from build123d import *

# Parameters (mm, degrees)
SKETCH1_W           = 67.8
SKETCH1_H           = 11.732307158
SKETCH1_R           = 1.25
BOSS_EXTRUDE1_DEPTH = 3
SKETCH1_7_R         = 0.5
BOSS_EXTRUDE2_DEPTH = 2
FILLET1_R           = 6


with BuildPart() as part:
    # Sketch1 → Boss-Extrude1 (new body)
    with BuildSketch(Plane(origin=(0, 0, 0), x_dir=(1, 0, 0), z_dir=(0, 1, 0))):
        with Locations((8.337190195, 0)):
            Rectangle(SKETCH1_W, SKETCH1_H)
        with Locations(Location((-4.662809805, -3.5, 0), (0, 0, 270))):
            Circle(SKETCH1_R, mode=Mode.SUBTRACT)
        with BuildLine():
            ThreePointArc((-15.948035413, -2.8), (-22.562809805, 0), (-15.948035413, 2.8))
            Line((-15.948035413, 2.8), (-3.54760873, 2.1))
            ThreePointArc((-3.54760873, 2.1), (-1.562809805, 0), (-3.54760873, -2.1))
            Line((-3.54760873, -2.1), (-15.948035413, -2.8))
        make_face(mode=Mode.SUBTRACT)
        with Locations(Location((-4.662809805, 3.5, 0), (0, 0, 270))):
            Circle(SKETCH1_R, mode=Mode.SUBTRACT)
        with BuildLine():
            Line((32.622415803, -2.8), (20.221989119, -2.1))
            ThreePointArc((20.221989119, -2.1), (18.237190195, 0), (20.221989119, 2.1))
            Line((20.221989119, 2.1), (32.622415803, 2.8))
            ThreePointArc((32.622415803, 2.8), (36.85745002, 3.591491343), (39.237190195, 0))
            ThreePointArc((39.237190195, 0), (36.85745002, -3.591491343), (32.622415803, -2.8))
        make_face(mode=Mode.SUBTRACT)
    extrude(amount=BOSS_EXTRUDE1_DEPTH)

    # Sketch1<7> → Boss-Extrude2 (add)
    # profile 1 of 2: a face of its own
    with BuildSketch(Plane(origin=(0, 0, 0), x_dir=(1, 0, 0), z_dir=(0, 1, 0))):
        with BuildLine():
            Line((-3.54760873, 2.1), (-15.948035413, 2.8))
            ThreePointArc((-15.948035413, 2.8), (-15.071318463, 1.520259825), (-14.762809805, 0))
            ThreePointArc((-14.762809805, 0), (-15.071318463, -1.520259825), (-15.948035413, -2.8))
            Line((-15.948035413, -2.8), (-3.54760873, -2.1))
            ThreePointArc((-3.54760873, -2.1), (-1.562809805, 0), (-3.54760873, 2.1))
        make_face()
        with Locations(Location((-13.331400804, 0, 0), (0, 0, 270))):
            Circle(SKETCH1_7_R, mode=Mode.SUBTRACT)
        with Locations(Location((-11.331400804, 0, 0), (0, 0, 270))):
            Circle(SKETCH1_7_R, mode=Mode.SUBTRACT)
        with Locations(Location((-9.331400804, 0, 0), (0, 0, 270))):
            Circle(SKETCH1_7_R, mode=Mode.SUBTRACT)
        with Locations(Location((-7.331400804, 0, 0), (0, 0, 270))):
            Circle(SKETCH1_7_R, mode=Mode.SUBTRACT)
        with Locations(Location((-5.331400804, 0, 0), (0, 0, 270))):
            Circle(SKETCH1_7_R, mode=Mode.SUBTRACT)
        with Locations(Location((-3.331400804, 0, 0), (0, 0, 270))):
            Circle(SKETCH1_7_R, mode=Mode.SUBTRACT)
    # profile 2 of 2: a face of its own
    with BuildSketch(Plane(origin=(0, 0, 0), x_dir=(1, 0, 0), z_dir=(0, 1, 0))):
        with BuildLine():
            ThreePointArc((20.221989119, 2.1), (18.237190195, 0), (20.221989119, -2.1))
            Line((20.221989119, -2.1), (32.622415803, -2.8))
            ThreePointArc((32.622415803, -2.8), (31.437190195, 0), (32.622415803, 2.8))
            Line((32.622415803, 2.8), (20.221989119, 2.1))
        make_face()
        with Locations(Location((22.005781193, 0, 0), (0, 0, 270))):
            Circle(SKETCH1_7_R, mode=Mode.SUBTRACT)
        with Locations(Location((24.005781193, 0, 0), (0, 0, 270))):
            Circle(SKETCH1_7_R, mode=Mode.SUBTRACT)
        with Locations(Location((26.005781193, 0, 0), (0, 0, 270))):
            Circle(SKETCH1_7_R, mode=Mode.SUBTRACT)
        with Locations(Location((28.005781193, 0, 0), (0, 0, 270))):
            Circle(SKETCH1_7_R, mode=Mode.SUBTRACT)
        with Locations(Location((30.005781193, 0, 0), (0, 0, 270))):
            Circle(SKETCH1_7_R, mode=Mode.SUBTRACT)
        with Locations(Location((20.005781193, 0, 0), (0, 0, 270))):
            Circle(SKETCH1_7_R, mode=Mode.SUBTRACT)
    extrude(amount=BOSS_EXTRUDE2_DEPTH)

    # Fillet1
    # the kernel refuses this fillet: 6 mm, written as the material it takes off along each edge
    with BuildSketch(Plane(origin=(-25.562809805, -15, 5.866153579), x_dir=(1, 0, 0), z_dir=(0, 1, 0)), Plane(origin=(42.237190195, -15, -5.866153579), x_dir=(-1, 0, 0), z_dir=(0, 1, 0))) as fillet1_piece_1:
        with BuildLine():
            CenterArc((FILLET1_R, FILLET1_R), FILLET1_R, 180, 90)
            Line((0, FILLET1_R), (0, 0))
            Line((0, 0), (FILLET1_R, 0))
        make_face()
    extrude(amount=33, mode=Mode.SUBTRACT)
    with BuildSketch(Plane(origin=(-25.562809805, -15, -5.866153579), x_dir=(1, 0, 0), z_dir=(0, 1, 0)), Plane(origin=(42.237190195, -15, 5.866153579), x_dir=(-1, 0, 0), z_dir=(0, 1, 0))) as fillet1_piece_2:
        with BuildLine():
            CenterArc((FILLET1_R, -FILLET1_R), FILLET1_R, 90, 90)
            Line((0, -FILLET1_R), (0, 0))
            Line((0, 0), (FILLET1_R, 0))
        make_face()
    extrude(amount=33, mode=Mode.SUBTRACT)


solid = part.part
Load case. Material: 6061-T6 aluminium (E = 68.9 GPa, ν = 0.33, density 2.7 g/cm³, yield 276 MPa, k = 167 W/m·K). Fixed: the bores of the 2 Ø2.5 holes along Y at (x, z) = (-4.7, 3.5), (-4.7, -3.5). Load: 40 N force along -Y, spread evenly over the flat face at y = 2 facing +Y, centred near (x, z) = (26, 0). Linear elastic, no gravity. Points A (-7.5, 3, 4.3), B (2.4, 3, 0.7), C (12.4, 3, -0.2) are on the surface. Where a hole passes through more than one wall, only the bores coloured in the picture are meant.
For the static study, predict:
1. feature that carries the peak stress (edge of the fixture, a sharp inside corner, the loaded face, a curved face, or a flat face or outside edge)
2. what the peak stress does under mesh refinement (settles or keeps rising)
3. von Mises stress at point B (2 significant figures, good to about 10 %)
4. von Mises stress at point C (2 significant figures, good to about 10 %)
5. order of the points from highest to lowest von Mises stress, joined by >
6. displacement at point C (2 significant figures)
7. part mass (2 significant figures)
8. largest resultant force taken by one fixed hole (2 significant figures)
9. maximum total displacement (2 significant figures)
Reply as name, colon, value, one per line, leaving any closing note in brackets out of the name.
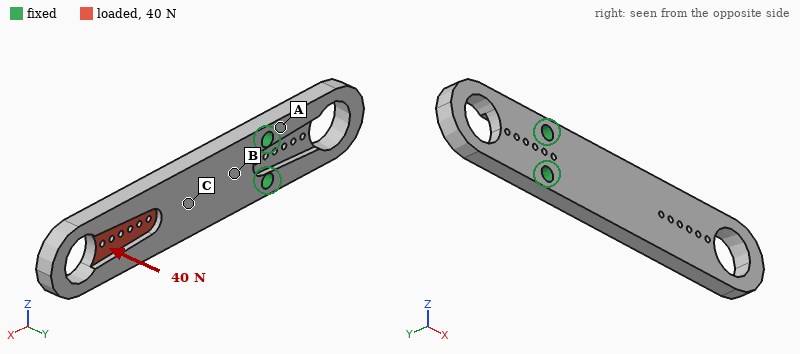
feature that carries the peak stress: edge of the fixture
what the peak stress does under mesh refinement: keeps rising
von Mises stress at point B: 48 MPa
von Mises stress at point C: 30 MPa
order of the points from highest to lowest von Mises stress, joined by >: B > C > A
displacement at point C: 0.078 mm
part mass: 5.0 g
largest resultant force taken by one fixed hole: 20 N
maximum total displacement: 0.37 mm
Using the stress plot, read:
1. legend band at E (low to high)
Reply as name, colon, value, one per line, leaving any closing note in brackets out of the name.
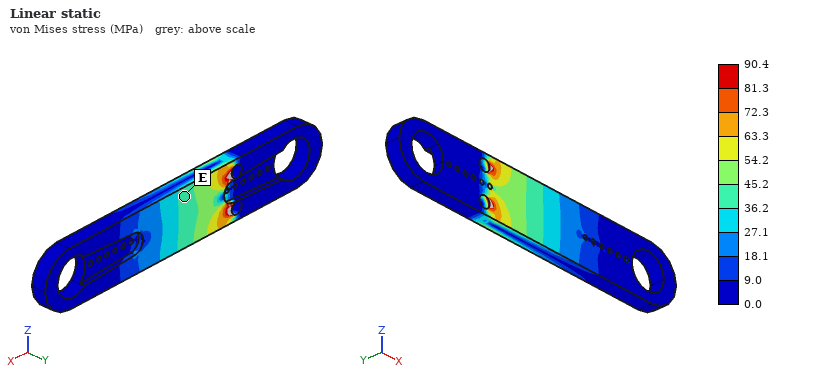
legend band at E: 36.2 to 45.2 MPa
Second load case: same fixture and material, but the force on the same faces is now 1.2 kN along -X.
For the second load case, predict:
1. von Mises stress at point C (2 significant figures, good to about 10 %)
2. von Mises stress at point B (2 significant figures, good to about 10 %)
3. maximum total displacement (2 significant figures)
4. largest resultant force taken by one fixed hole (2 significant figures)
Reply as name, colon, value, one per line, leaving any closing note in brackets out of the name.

von Mises stress at point C: 66 MPa
von Mises stress at point B: 63 MPa
maximum total displacement: 0.36 mm
largest resultant force taken by one fixed hole: 610 N
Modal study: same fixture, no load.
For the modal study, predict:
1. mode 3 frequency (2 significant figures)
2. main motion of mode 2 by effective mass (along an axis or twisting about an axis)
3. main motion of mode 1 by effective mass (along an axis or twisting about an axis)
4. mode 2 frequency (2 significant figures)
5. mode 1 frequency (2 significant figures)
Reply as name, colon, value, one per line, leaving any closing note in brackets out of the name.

mode 3 frequency: 6800 Hz
main motion of mode 2 by effective mass: along Z
main motion of mode 1 by effective mass: along Y
mode 2 frequency: 5200 Hz
mode 1 frequency: 1400 Hz
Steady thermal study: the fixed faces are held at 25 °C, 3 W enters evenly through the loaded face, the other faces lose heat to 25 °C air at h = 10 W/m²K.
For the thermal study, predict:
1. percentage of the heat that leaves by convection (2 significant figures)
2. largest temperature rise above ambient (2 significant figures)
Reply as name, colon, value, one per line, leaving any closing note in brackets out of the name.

percentage of the heat that leaves by convection: 4.4 %
largest temperature rise above ambient: 16 K
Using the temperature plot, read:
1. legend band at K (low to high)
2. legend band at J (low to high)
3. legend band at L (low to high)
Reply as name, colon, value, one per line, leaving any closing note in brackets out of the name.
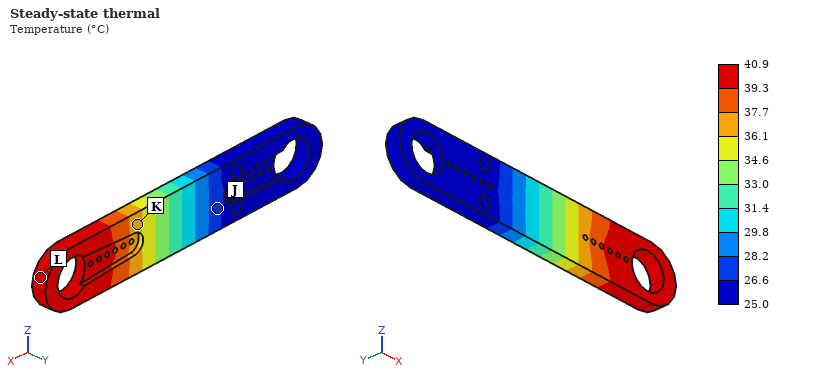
legend band at K: 36.1 to 37.7 °C
legend band at J: 26.6 to 28.2 °C
legend band at L: 39.3 to 40.9 °C
